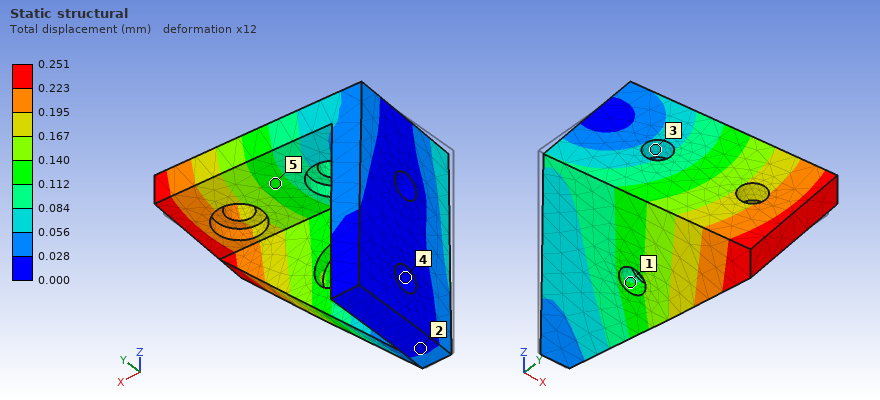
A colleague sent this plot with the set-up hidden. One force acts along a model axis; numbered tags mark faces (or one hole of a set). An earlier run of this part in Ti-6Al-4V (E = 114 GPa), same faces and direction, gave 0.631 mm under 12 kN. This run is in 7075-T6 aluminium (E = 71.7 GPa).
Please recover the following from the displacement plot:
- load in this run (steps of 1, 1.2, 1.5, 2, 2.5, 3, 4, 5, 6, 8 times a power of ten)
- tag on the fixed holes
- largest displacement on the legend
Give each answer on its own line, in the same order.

3 kN
4
0.251 mm
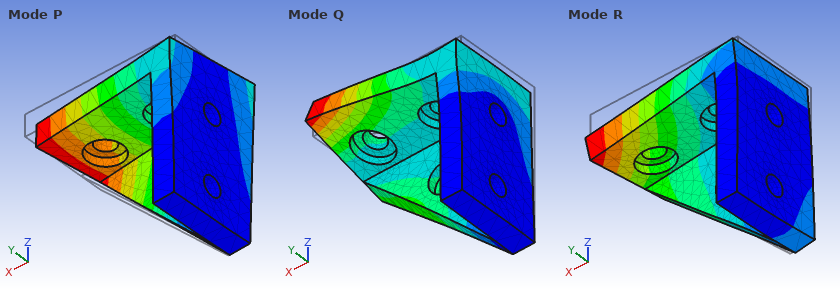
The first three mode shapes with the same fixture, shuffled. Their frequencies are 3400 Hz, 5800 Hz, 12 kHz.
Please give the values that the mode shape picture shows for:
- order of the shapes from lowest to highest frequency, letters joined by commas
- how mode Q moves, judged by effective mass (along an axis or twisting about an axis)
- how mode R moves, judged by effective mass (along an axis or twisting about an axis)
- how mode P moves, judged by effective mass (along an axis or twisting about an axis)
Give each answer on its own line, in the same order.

P, R, Q
along X
along Z
along Y
